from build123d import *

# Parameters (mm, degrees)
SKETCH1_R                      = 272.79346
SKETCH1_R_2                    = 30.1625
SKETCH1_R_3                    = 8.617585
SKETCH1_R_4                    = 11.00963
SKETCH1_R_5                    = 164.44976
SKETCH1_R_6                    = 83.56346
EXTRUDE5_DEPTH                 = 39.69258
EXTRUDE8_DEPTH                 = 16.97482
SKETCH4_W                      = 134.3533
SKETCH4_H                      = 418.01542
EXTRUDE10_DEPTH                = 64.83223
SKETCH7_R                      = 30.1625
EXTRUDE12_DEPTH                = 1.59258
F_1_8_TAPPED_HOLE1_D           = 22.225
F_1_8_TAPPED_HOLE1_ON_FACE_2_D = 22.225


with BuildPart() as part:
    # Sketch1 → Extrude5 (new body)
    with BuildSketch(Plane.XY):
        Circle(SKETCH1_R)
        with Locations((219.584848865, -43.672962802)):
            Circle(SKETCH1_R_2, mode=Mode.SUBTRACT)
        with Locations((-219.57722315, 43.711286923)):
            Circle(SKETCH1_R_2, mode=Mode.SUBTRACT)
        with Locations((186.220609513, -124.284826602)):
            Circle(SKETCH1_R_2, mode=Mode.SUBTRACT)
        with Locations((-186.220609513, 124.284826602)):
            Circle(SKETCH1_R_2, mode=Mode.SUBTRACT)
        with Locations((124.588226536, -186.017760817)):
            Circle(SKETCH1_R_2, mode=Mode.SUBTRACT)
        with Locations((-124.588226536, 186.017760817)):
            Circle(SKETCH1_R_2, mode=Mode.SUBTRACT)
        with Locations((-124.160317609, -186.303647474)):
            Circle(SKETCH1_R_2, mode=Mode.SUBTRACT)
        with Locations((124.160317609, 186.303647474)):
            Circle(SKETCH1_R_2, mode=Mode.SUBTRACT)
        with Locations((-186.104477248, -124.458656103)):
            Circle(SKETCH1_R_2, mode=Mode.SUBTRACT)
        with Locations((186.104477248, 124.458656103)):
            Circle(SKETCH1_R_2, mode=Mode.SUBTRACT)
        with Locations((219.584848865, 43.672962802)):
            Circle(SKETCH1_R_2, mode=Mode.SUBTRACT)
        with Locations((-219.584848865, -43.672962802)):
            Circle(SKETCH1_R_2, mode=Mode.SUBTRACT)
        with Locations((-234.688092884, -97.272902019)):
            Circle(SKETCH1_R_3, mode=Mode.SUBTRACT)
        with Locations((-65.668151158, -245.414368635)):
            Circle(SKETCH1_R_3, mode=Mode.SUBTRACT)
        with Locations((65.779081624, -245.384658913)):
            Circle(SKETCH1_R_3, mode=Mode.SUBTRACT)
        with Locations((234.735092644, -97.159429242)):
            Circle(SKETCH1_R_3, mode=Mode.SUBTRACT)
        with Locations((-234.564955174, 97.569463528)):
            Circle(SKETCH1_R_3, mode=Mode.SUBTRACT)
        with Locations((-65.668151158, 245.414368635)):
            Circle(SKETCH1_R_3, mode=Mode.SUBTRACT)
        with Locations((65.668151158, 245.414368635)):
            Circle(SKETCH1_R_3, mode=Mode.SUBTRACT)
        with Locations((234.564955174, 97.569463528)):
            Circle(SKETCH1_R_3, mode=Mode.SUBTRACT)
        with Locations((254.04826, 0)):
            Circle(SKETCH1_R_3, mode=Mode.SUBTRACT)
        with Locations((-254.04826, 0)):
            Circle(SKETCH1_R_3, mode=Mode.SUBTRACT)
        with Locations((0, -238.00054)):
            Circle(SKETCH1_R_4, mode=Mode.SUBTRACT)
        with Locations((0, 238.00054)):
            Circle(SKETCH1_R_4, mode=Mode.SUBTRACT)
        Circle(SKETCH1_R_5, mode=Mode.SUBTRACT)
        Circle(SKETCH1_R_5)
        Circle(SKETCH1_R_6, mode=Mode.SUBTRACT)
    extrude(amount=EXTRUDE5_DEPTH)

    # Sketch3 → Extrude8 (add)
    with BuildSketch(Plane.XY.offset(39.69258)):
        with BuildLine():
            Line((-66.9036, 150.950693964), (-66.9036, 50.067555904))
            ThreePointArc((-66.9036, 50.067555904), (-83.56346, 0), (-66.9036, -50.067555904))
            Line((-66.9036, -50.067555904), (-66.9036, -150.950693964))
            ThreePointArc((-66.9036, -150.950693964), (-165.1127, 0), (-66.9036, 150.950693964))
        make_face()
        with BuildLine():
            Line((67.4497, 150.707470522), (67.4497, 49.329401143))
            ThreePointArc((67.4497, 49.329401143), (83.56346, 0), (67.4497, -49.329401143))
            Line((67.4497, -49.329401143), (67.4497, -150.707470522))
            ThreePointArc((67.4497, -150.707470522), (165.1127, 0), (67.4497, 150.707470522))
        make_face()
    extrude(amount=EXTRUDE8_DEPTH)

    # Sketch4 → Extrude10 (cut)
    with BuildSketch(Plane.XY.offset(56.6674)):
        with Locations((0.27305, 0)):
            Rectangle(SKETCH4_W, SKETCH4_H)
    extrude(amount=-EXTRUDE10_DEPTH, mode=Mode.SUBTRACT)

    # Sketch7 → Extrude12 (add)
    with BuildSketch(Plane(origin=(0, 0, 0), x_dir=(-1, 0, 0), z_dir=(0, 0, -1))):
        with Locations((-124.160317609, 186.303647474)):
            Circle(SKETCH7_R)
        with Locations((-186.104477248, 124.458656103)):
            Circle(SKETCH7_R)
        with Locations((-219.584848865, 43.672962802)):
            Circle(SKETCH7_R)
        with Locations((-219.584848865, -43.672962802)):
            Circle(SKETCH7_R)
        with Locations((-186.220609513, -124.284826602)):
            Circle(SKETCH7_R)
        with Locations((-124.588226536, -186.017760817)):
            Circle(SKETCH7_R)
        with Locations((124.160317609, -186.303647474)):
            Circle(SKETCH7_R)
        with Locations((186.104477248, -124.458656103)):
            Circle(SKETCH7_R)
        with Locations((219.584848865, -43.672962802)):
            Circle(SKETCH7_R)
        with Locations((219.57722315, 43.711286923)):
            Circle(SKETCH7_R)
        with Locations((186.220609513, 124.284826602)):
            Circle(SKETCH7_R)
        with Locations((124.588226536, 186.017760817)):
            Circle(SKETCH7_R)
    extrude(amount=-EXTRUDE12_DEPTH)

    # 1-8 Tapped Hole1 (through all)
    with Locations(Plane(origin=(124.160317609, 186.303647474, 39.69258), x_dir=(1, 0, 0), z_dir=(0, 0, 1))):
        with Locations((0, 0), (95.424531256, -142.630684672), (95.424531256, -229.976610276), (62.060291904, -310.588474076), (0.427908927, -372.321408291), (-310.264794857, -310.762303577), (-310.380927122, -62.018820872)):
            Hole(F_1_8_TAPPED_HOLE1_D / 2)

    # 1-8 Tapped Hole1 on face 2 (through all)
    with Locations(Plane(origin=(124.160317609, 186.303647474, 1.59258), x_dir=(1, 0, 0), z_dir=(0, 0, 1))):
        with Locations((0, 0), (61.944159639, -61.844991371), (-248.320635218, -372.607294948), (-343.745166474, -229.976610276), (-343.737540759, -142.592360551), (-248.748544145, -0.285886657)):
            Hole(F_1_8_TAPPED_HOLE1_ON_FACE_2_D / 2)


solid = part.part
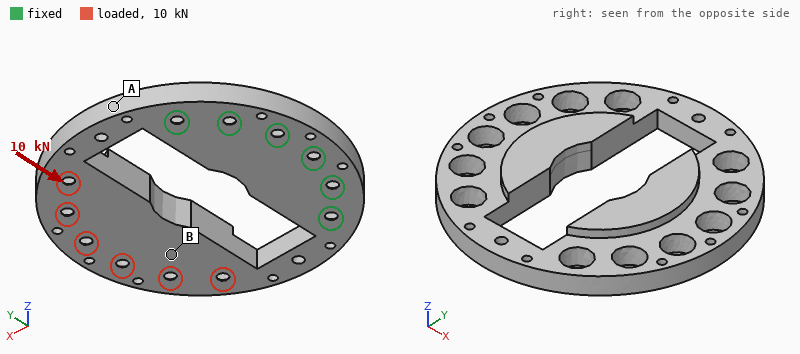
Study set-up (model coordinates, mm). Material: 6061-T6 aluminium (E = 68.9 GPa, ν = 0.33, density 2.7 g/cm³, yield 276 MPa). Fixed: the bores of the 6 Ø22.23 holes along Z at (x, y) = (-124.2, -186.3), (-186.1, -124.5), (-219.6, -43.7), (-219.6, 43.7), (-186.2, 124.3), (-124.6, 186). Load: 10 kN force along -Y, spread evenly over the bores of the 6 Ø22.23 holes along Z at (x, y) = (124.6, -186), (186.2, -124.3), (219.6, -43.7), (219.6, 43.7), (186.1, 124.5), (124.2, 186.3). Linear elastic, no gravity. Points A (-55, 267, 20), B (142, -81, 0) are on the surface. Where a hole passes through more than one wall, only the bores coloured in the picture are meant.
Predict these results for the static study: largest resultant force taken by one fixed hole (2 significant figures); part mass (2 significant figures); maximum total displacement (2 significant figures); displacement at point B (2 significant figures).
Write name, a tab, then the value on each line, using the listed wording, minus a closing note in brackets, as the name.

largest resultant force taken by one fixed hole	7.4 kN
part mass	17 kg
maximum total displacement	0.30 mm
displacement at point B	0.26 mm
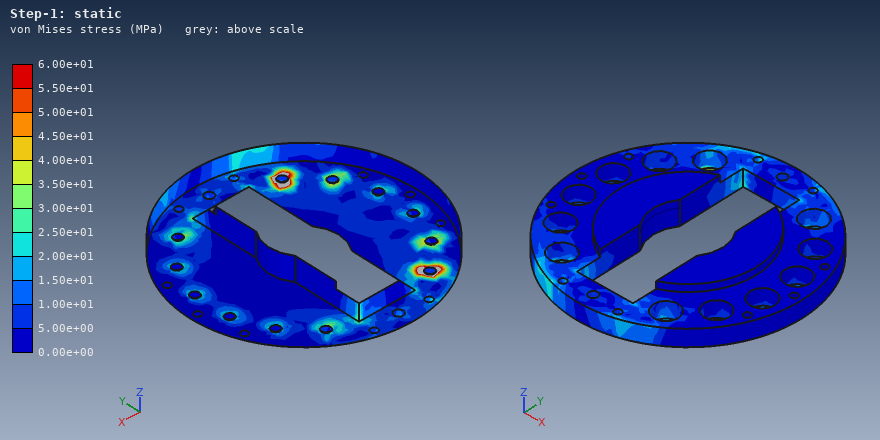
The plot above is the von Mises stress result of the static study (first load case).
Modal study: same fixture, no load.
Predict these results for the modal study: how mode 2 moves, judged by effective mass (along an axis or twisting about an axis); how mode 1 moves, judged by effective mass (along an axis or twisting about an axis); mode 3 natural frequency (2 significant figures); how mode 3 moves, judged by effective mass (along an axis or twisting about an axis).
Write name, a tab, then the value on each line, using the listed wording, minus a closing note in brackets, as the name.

how mode 2 moves, judged by effective mass	twisting about X
how mode 1 moves, judged by effective mass	along Z
mode 3 natural frequency	360 Hz
how mode 3 moves, judged by effective mass	along Y
